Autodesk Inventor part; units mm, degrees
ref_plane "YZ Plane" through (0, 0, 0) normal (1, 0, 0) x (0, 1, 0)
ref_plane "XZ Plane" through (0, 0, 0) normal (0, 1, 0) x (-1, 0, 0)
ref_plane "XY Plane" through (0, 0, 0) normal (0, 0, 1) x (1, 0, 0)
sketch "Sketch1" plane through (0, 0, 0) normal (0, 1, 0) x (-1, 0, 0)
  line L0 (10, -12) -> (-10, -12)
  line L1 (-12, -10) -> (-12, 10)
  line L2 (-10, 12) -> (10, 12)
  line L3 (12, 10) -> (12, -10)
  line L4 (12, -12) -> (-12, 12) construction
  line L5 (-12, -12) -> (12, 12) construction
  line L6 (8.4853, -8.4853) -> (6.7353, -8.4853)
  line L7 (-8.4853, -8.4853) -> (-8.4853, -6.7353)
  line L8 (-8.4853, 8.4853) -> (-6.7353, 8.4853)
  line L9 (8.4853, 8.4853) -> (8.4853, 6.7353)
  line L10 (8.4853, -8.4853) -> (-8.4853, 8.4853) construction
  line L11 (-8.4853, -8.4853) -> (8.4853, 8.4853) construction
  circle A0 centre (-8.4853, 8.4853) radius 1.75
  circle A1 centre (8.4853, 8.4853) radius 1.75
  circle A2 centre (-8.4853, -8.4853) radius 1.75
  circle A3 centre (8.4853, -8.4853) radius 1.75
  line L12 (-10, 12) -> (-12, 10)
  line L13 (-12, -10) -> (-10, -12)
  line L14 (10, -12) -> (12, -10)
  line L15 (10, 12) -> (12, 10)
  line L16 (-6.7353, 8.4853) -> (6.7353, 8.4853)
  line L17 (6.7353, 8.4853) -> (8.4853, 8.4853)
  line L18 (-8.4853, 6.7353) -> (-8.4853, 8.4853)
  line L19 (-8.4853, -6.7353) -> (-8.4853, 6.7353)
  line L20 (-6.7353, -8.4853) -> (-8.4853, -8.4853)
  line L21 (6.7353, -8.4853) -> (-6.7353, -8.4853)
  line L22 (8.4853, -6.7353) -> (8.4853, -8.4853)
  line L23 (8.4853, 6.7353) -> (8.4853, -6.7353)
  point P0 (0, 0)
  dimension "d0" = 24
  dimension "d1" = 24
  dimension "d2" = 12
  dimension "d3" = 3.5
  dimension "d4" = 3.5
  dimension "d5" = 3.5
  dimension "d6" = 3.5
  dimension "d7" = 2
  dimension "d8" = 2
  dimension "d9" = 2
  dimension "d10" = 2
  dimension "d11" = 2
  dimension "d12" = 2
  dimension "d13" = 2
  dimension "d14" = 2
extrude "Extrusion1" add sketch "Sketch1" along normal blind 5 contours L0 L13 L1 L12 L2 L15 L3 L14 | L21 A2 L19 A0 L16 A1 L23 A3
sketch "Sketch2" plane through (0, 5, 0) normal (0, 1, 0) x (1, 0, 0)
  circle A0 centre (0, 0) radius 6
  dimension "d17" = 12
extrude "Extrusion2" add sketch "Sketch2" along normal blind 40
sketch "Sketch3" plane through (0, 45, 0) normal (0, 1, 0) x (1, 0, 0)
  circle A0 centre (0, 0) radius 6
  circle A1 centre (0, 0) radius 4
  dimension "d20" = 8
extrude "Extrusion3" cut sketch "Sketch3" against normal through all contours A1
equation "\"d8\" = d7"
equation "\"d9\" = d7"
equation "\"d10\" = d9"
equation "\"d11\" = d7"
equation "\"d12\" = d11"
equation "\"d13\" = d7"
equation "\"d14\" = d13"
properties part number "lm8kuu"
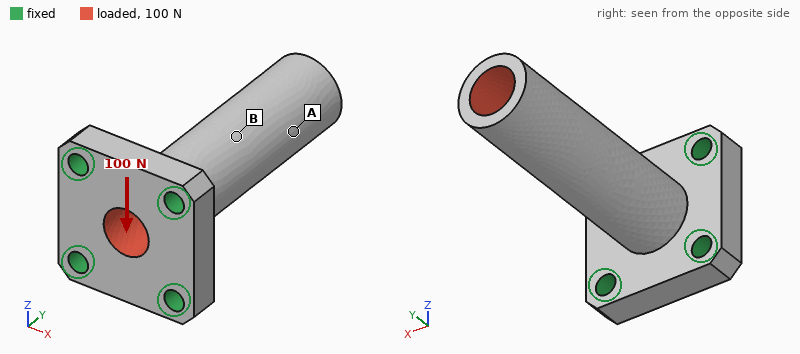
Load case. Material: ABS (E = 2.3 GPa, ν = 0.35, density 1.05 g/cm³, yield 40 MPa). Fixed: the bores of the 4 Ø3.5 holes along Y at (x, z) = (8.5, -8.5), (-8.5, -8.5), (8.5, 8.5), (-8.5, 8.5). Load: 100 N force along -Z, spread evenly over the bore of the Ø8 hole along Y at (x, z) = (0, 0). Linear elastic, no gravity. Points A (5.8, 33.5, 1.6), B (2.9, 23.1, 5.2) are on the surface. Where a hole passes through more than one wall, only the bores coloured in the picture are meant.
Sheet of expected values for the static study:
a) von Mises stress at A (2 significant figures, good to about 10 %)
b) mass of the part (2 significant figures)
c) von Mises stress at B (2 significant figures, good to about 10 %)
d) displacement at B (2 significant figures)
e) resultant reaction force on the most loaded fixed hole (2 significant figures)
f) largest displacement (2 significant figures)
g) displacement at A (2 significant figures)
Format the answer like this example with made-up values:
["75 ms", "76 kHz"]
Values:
["1.2 MPa", "5.2 g", "3.6 MPa", "0.27 mm", "76 N", "0.66 mm", "0.44 mm"]
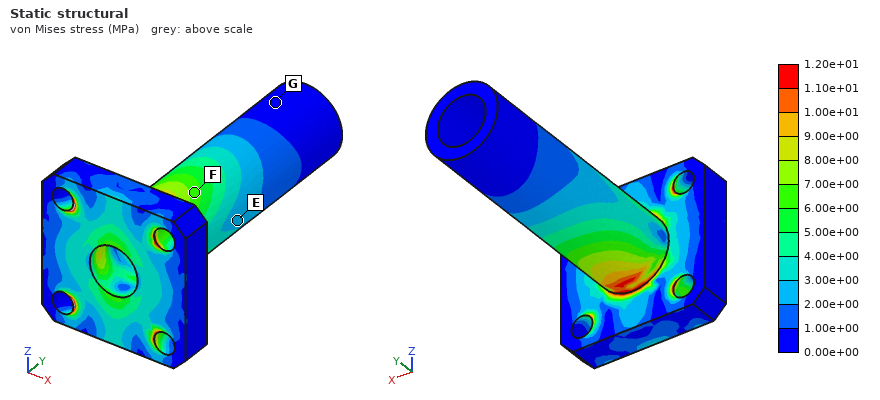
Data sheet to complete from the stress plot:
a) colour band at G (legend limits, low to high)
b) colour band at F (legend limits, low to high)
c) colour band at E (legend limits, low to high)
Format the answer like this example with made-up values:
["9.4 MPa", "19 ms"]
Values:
["0.00e+00 to 1.00e+00 MPa", "6.00e+00 to 7.00e+00 MPa", "2.00e+00 to 3.00e+00 MPa"]
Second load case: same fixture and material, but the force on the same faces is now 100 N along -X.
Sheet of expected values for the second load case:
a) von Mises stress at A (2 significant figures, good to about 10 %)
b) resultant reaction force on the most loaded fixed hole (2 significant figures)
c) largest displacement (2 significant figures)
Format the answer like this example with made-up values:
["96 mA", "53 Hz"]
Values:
["1.1 MPa", "76 N", "0.66 mm"]
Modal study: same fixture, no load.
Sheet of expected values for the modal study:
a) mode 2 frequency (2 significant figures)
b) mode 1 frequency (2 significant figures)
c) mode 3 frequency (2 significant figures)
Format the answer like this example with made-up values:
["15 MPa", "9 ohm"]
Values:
["1400 Hz", "1400 Hz", "5400 Hz"]
